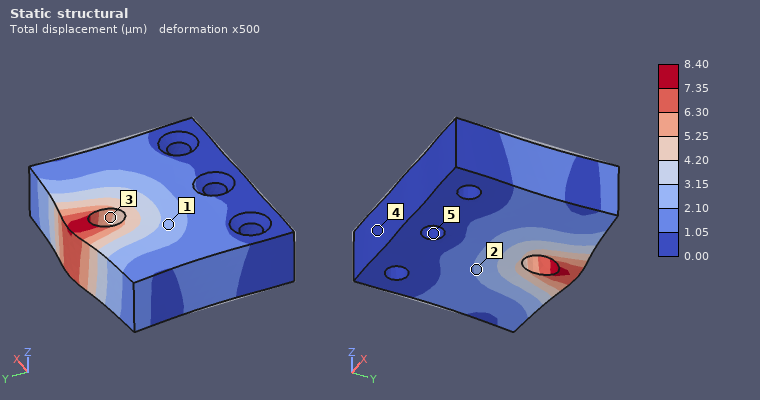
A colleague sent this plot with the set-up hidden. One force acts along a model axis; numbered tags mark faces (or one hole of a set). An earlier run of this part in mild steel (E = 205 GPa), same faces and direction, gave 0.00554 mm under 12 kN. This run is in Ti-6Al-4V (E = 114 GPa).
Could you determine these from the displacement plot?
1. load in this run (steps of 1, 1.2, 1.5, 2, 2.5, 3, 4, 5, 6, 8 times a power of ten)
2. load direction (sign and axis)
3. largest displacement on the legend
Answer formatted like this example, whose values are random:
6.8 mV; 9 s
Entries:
10 kN; +Y; 8.40 µm
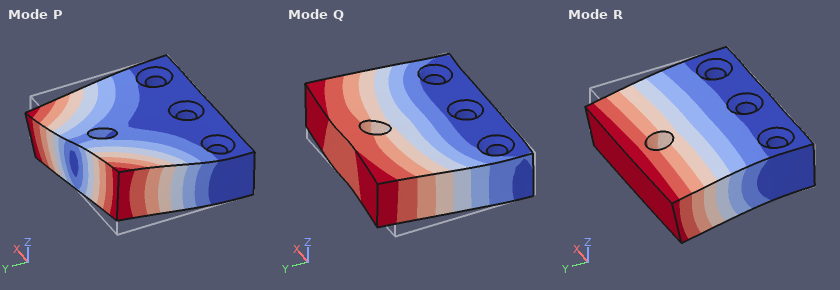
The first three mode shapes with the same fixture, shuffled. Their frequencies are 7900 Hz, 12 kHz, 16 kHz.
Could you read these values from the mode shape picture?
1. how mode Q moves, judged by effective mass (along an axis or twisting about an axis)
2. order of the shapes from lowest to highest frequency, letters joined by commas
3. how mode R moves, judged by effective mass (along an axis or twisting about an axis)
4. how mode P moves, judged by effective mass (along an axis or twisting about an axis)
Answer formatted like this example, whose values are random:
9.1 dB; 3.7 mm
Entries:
along X; R, P, Q; along Z; twisting about Y
